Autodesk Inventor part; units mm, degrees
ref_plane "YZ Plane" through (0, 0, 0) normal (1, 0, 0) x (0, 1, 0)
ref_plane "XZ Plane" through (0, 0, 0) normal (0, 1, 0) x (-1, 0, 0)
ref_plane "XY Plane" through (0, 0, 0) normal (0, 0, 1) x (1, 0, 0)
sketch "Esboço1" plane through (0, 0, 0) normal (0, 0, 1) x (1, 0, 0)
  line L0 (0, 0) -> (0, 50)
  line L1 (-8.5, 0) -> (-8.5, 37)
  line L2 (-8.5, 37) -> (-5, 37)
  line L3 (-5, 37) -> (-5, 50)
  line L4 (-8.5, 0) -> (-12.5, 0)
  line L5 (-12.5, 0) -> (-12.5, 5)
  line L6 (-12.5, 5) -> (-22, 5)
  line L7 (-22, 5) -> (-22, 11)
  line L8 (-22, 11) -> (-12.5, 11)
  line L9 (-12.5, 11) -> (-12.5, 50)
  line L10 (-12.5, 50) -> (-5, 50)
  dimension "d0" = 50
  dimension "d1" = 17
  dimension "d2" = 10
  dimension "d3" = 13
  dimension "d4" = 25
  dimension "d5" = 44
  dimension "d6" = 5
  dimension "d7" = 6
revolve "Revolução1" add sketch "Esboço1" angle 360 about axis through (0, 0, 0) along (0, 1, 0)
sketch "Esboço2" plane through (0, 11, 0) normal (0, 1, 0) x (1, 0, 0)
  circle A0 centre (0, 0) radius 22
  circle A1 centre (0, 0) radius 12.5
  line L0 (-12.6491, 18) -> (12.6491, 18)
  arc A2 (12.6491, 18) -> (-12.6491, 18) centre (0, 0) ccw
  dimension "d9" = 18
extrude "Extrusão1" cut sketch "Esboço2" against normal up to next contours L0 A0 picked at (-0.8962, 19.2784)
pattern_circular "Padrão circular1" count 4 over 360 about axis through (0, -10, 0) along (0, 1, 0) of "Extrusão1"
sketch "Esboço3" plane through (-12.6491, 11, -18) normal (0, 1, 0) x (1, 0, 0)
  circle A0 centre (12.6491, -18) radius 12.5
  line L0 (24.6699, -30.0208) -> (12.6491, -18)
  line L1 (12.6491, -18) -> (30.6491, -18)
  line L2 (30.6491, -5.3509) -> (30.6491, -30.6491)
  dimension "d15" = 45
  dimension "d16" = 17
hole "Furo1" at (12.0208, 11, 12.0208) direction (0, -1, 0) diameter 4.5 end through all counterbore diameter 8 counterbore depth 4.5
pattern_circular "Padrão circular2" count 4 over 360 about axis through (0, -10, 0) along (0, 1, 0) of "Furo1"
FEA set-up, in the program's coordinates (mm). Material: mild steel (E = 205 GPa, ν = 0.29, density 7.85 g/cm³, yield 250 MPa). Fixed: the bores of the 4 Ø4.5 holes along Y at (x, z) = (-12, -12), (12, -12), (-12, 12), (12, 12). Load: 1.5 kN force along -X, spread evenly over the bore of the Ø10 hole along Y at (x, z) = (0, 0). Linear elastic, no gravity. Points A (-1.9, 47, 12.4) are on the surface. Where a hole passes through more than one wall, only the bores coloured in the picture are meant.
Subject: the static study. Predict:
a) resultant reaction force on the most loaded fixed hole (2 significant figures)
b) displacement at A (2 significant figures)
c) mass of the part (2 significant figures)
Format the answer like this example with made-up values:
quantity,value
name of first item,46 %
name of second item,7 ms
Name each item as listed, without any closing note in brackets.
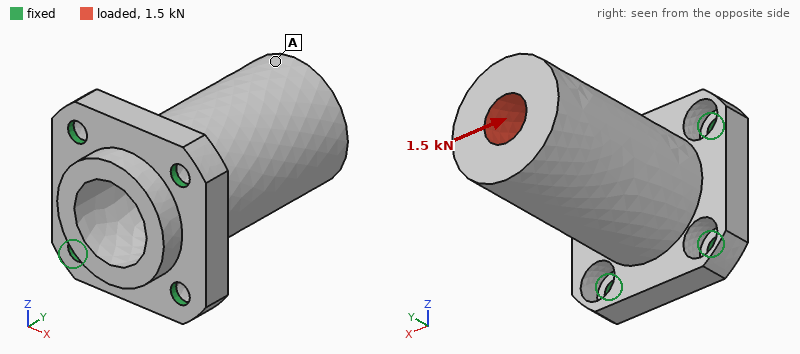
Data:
quantity,value
resultant reaction force on the most loaded fixed hole,1.3 kN
displacement at A,28 µm
mass of the part,150 g
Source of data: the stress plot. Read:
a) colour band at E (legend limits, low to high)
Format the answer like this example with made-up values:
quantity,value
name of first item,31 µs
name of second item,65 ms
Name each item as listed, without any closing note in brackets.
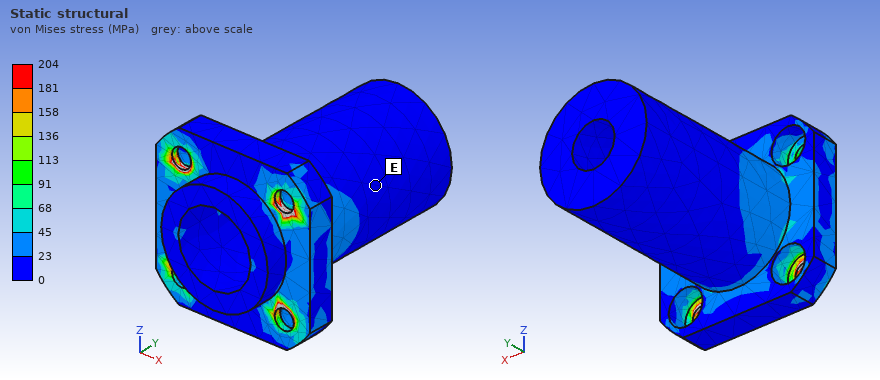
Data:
quantity,value
colour band at E,0 to 23 MPa
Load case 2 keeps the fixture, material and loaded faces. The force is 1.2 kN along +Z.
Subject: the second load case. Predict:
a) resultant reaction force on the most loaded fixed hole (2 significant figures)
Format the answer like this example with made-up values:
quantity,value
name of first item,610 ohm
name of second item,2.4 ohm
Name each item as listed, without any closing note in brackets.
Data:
quantity,value
resultant reaction force on the most loaded fixed hole,1.1 kN
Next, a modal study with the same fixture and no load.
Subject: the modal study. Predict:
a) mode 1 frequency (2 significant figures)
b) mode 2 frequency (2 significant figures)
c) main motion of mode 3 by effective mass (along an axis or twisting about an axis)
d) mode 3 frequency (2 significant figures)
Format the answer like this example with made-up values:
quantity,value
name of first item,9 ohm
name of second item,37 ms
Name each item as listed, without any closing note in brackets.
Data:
quantity,value
mode 1 frequency,5000 Hz
mode 2 frequency,5000 Hz
main motion of mode 3 by effective mass,along Y
mode 3 frequency,13 kHz
